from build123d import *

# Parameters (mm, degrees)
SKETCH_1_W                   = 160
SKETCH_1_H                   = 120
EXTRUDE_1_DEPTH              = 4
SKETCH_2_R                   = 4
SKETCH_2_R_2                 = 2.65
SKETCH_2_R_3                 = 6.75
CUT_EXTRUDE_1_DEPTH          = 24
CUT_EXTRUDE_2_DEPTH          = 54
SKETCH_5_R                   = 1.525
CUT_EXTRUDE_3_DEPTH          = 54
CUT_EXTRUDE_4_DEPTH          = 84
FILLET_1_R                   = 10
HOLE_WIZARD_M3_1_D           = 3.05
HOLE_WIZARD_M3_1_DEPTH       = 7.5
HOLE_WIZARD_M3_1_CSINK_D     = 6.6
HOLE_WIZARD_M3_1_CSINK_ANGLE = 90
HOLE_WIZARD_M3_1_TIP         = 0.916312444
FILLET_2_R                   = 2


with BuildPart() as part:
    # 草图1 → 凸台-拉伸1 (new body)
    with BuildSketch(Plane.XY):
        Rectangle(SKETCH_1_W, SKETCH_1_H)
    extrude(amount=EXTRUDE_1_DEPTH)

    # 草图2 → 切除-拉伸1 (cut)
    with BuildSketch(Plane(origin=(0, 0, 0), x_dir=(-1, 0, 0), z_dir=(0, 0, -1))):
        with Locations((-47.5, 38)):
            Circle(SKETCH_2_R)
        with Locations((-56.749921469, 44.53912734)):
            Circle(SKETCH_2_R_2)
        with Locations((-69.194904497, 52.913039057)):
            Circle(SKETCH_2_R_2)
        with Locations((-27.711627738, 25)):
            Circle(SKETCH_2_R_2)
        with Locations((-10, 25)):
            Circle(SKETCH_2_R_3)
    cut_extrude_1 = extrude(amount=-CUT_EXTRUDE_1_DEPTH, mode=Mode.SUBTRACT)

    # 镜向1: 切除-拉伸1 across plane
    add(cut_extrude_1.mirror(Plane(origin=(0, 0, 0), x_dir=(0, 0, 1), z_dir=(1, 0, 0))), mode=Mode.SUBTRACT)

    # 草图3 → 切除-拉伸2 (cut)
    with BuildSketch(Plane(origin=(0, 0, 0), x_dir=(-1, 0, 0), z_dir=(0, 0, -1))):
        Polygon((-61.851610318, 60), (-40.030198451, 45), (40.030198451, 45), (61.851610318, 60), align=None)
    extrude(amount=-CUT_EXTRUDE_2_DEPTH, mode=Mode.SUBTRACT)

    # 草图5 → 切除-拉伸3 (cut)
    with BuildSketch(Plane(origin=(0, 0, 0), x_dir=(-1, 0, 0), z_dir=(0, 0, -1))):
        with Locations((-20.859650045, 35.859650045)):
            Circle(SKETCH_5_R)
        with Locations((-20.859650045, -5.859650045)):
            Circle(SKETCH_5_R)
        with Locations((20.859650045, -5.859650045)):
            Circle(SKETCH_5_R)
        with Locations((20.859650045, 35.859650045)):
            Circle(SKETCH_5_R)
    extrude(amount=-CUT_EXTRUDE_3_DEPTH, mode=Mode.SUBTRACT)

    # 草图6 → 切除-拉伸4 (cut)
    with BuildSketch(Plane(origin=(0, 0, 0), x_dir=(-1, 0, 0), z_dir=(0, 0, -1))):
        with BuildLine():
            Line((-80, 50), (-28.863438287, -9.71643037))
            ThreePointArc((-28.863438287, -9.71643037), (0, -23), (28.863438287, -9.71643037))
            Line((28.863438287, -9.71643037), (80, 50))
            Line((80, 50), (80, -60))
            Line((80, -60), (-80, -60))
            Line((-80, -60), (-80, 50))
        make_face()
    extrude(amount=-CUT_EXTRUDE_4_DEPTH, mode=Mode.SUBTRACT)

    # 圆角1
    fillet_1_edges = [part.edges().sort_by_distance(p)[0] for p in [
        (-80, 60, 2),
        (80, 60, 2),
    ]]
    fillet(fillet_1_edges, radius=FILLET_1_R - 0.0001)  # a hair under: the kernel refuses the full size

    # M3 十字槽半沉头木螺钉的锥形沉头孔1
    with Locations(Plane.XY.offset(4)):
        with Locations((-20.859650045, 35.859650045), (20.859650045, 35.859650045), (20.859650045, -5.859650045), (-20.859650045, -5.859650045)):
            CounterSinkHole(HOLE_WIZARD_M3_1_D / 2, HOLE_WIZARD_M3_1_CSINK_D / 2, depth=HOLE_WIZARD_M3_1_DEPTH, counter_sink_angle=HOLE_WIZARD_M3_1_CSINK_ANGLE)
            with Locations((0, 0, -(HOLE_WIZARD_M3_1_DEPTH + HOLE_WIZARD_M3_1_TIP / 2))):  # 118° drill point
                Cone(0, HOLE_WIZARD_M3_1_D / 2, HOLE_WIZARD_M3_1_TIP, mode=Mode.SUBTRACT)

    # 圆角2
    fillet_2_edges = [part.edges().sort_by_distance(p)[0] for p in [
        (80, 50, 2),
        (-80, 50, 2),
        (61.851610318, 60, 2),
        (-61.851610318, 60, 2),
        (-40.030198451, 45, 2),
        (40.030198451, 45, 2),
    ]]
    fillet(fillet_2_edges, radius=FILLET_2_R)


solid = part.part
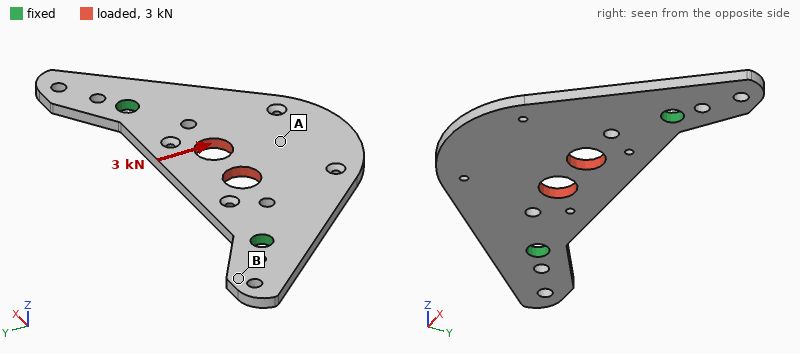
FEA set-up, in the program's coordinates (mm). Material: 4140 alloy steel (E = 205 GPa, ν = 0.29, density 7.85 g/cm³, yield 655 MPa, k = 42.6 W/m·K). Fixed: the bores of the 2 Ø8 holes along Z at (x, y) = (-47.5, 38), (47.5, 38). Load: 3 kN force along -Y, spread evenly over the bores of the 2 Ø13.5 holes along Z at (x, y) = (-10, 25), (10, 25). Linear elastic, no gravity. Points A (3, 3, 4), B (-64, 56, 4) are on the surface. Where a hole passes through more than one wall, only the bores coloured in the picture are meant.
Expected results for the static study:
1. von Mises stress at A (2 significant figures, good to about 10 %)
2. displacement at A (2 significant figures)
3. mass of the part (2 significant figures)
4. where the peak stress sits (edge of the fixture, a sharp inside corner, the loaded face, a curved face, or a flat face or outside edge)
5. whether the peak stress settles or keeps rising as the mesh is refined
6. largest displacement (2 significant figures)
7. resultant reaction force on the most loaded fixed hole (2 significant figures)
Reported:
15 MPa
5.8 µm
200 g
edge of the fixture
keeps rising
7.9 µm
1.7 kN
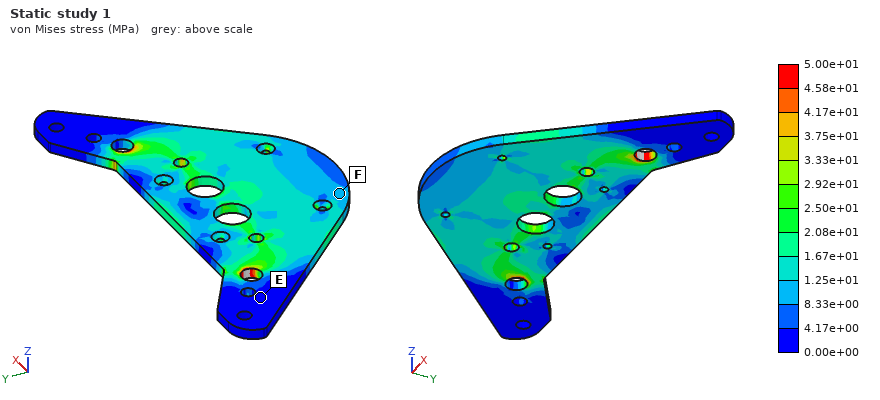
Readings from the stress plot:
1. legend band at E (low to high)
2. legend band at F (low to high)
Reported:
0.00e+00 to 4.17e+00 MPa
8.33e+00 to 1.25e+01 MPa
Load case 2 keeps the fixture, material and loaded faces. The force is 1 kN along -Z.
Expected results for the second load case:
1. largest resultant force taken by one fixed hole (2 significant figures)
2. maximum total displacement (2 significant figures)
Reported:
500 N
0.17 mm
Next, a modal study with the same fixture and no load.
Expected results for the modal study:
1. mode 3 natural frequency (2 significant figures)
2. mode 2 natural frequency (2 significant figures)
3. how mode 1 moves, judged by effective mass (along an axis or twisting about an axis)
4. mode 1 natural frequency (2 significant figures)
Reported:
2800 Hz
2800 Hz
along Z
900 Hz
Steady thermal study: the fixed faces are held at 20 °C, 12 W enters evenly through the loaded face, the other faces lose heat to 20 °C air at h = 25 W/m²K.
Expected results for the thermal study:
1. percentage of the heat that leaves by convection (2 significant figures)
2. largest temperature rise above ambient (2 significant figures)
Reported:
41 %
35 K
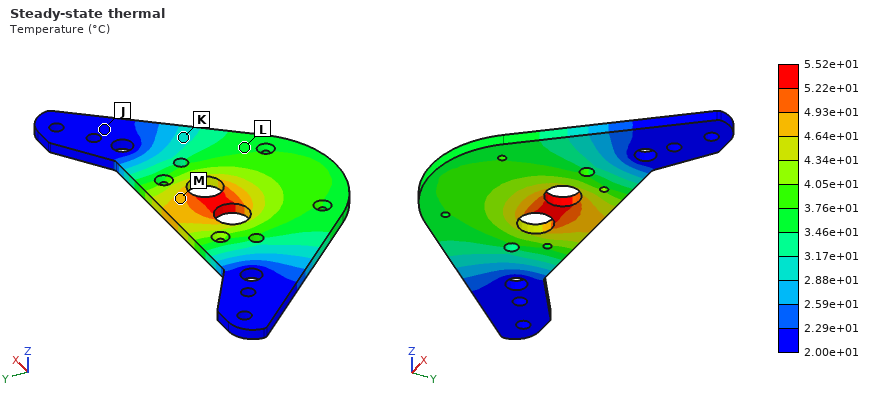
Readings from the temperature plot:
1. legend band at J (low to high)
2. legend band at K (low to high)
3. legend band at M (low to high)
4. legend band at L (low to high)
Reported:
2.00e+01 to 2.29e+01 °C
2.88e+01 to 3.17e+01 °C
4.64e+01 to 4.93e+01 °C
3.46e+01 to 3.76e+01 °C
